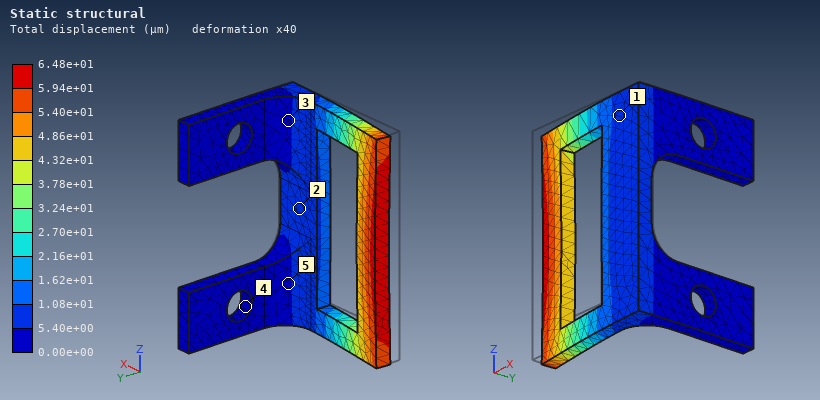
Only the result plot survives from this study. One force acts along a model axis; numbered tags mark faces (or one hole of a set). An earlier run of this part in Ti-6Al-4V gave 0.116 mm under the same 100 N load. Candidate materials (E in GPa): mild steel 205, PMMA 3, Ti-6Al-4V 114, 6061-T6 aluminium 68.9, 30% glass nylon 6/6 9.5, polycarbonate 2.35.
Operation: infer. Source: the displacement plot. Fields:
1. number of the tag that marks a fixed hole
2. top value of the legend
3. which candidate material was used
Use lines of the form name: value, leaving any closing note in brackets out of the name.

number of the tag that marks a fixed hole: 4
top value of the legend: 6.48e+01 µm
which candidate material was used: mild steel
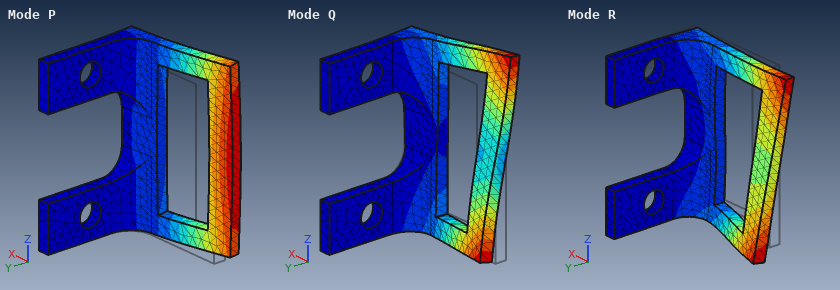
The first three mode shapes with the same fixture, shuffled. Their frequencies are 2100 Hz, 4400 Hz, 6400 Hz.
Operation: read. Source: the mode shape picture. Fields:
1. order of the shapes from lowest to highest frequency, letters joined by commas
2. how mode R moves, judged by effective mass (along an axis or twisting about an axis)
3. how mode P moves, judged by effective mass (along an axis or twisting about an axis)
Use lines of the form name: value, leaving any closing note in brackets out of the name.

order of the shapes from lowest to highest frequency, letters joined by commas: P, Q, R
how mode R moves, judged by effective mass: along Z
how mode P moves, judged by effective mass: along Y
